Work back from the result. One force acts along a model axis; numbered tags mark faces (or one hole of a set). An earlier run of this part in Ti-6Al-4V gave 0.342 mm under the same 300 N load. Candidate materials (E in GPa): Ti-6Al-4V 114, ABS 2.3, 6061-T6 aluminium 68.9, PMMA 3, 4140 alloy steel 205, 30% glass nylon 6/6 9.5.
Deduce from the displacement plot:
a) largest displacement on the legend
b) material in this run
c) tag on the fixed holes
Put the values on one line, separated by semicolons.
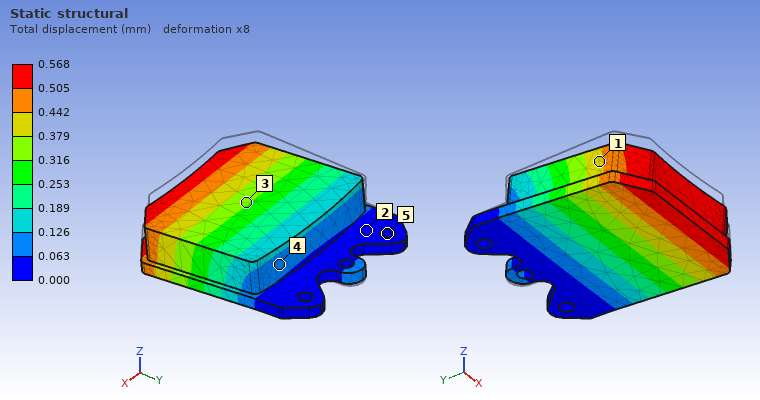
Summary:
0.568 mm; 6061-T6 aluminium; 5
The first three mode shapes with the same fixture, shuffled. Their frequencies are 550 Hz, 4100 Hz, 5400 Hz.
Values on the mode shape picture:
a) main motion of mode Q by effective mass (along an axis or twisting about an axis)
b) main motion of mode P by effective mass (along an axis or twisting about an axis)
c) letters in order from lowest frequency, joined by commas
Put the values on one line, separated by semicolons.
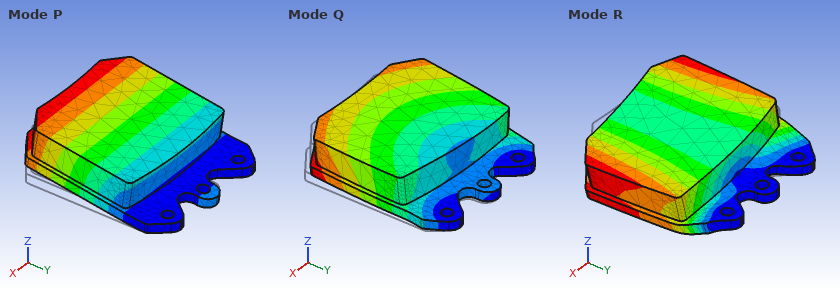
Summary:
along X; along Z; P, R, Q
